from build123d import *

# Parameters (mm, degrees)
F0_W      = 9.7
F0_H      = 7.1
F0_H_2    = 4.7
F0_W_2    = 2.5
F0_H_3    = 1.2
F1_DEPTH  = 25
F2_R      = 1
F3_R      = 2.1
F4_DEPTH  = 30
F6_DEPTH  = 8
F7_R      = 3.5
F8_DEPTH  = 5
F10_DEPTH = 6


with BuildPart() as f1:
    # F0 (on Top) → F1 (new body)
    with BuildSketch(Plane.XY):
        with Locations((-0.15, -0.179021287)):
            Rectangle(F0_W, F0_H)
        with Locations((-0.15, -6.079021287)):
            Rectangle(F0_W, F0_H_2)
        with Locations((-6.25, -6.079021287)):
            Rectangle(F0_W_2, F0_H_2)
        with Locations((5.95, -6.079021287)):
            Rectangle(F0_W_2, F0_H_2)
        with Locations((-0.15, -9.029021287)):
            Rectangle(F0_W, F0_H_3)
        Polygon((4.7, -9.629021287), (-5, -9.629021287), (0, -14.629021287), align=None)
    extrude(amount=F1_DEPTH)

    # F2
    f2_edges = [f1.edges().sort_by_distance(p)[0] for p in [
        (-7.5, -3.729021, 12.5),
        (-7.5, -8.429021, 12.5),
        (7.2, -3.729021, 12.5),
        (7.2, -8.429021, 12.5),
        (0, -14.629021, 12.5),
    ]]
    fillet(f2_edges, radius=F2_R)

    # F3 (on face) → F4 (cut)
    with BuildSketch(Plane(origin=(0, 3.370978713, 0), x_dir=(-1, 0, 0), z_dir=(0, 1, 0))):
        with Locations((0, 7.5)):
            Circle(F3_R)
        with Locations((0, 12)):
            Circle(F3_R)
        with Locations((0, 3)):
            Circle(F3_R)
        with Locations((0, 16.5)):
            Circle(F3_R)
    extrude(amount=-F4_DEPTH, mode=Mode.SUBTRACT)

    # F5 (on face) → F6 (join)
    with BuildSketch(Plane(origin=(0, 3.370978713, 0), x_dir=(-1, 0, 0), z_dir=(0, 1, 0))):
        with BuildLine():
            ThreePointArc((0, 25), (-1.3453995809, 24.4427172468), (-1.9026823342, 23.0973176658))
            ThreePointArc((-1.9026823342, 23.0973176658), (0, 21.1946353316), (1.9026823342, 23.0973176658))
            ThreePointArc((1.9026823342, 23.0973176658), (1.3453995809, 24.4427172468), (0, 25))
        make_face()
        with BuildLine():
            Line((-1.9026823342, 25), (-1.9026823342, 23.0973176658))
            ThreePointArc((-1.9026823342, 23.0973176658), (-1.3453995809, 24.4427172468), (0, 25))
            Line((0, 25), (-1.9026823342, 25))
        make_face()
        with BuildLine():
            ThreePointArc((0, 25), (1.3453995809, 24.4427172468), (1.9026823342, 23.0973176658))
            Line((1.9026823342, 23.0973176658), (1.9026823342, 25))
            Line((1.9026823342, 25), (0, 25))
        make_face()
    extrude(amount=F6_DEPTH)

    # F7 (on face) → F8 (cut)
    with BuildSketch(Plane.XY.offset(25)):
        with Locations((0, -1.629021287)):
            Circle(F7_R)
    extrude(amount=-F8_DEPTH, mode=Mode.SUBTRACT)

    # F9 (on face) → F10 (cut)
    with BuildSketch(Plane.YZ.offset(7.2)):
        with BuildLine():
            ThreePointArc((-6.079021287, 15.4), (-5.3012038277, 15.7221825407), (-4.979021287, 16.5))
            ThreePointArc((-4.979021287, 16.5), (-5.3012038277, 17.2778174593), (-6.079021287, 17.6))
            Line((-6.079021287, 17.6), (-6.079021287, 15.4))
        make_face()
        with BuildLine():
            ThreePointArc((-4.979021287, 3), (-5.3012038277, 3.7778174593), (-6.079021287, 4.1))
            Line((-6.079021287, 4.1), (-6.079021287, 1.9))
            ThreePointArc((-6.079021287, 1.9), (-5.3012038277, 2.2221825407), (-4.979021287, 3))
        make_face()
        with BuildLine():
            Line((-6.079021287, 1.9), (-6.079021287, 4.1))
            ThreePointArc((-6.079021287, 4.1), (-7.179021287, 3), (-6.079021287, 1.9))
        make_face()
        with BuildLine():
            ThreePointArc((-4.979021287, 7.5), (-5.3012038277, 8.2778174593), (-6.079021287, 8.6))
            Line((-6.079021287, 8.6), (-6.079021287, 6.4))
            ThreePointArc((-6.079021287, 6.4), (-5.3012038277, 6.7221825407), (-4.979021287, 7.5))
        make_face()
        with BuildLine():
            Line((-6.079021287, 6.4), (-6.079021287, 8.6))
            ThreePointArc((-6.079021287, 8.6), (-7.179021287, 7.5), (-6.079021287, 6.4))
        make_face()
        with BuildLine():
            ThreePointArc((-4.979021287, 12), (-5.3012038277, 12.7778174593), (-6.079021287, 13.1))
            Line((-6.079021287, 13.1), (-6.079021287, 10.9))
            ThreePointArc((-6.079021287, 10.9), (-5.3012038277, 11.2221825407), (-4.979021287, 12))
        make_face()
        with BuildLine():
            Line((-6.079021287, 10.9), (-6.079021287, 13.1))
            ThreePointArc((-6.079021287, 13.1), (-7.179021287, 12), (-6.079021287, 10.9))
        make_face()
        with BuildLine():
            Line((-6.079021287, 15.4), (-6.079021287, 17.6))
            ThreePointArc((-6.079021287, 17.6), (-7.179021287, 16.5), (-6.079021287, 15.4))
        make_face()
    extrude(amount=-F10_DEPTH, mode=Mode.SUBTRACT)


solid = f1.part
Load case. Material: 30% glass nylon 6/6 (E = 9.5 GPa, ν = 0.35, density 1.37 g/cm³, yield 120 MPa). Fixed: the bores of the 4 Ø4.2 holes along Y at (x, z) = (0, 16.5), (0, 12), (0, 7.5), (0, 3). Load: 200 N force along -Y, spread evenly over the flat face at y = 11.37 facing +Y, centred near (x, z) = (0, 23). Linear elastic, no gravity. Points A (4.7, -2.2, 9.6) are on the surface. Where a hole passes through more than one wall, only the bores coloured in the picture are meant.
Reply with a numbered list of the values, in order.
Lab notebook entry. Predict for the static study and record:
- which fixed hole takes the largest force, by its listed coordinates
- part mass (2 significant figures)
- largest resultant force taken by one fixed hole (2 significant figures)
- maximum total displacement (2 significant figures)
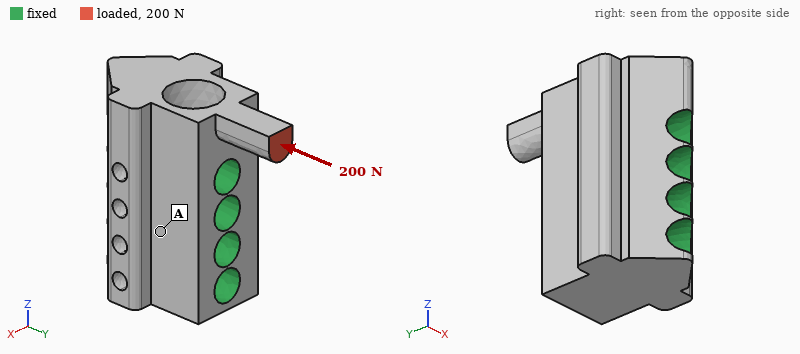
1. (0, 16.5)
2. 4.4 g
3. 200 N
4. 65 µm
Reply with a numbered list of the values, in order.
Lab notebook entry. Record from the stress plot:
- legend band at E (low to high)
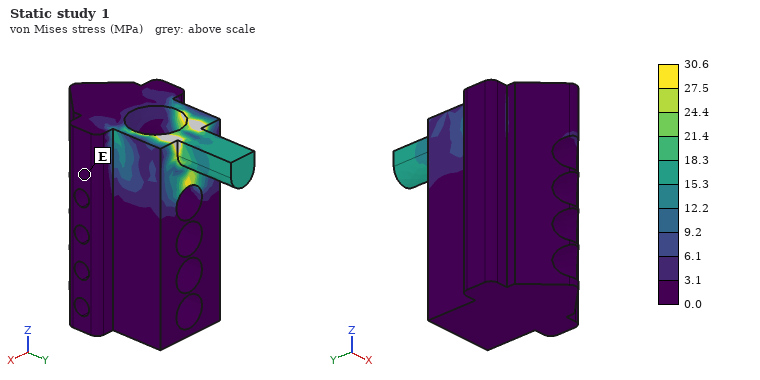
1. 0.0 to 3.1 MPa
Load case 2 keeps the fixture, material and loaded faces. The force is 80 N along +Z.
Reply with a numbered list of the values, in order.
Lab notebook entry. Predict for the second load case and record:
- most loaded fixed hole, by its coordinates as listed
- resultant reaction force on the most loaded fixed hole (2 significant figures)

1. (0, 16.5)
2. 92 N
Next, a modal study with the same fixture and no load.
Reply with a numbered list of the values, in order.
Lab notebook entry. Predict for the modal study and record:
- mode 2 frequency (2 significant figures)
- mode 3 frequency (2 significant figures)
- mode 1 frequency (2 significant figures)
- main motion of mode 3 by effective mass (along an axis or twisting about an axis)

1. 14 kHz
2. 32 kHz
3. 13 kHz
4. along X
